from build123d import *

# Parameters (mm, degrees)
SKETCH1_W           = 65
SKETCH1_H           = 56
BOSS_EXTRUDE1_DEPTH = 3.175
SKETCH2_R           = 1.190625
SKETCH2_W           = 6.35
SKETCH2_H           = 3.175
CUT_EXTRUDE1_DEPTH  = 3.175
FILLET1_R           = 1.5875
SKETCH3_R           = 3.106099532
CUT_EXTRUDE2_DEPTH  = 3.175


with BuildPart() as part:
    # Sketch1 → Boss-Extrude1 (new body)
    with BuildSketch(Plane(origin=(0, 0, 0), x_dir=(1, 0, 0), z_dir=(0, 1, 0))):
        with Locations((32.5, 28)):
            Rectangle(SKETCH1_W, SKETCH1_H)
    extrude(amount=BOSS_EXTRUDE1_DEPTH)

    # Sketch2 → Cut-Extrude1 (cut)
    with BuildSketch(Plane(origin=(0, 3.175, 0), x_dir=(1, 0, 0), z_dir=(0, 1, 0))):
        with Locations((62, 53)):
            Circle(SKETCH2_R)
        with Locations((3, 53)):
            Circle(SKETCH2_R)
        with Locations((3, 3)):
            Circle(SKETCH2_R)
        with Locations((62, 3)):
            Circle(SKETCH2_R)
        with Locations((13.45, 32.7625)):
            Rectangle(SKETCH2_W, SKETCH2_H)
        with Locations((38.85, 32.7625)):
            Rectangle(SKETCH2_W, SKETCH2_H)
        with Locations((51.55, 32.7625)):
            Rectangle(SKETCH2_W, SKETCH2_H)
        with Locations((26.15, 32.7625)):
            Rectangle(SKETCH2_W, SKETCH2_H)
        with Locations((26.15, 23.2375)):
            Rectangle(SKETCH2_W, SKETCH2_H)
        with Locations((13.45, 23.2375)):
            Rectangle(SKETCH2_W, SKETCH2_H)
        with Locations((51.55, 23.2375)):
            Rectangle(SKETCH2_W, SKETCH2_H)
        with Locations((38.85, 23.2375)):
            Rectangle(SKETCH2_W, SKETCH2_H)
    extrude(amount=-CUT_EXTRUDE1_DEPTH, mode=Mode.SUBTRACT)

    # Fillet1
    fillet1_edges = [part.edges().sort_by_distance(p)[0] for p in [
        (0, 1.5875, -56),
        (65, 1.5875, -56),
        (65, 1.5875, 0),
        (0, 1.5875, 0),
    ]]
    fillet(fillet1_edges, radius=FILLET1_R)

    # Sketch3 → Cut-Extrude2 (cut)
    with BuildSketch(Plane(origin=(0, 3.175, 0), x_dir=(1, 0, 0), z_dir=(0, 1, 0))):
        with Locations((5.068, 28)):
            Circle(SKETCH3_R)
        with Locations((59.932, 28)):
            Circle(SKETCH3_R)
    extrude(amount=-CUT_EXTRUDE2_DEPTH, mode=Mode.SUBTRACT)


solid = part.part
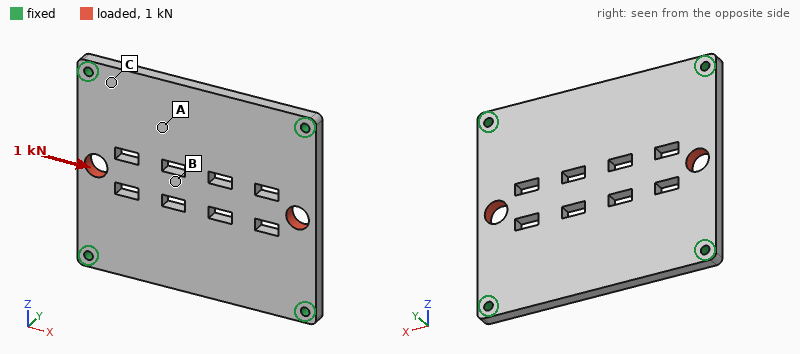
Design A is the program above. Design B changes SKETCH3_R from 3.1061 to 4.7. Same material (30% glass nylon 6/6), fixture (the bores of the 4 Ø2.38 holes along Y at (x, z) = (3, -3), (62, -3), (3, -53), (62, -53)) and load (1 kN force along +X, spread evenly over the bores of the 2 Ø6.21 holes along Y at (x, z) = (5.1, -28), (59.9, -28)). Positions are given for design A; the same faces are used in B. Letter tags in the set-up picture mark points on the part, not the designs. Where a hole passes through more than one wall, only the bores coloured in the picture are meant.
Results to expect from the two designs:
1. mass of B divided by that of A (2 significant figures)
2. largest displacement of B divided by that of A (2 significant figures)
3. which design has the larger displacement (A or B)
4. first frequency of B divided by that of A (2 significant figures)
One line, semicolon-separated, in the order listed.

0.98; 1.8; B; 0.99
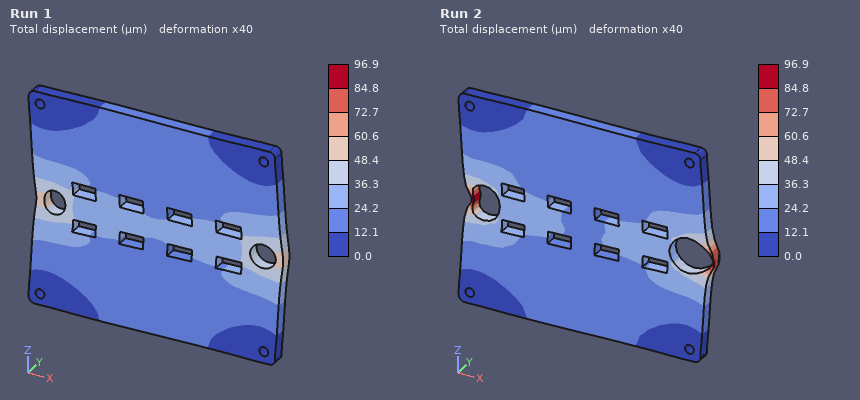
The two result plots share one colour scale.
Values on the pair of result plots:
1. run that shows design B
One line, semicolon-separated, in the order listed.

Run 2
